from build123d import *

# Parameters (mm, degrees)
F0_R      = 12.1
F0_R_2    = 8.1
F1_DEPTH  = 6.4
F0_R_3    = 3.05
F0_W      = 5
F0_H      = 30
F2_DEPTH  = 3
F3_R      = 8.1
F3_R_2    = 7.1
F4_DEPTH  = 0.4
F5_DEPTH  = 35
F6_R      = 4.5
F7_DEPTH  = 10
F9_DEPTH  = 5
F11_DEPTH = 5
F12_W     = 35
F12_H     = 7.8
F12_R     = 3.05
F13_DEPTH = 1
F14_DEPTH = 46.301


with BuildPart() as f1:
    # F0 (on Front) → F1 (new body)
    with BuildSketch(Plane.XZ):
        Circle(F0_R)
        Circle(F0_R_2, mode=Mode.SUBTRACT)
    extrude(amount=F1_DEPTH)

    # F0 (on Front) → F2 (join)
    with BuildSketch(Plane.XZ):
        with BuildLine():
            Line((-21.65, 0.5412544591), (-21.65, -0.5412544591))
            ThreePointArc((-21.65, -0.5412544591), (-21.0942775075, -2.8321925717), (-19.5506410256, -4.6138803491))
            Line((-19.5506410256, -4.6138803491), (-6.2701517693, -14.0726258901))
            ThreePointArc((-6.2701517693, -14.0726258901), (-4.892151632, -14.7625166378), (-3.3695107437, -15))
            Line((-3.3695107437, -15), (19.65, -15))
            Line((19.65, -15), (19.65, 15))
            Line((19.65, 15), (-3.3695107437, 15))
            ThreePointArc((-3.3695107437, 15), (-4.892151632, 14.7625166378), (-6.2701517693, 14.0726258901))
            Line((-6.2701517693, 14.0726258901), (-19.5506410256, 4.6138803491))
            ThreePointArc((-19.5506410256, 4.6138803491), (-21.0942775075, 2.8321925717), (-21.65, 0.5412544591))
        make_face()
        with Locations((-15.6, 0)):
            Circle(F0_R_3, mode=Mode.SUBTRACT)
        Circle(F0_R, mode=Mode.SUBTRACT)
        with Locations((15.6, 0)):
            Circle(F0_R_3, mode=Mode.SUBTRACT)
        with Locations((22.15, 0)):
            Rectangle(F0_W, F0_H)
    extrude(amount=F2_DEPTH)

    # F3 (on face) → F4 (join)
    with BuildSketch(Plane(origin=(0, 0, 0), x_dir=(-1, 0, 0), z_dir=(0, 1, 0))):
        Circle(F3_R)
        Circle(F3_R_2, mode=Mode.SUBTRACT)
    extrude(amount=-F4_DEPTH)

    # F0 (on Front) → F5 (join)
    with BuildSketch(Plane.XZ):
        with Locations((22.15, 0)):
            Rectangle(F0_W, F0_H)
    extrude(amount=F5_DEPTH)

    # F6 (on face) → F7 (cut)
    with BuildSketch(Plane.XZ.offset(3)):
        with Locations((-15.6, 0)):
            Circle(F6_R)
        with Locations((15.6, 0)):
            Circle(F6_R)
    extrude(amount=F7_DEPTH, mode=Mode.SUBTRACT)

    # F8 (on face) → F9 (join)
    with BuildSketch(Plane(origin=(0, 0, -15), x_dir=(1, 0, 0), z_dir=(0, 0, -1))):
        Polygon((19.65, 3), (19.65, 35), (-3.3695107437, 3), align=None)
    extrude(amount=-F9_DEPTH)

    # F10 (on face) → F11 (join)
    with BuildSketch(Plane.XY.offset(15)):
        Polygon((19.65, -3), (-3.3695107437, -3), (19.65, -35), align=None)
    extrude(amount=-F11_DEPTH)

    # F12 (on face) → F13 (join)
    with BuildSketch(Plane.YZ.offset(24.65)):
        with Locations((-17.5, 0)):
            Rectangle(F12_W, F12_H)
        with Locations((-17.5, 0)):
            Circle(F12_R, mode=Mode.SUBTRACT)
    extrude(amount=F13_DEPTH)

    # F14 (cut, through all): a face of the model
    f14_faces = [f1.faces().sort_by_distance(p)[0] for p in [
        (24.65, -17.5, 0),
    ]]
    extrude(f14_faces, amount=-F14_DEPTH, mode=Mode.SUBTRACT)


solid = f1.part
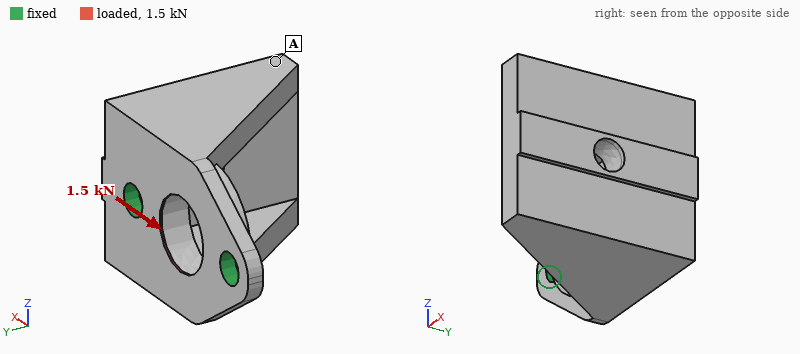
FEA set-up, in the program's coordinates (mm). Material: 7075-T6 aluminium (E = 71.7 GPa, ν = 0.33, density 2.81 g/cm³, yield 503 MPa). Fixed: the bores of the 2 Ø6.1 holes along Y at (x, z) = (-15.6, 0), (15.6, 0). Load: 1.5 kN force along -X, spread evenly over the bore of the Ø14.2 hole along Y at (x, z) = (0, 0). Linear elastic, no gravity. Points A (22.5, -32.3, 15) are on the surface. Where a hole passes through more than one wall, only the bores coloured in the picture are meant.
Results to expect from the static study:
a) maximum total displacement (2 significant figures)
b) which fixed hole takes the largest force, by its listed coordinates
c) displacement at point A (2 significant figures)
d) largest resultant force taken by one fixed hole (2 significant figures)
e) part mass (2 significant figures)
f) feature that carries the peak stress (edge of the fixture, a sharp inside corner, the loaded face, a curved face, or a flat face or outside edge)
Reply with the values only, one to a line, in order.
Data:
6.5 µm
(15.6, 0)
1.2 µm
810 N
34 g
the loaded face
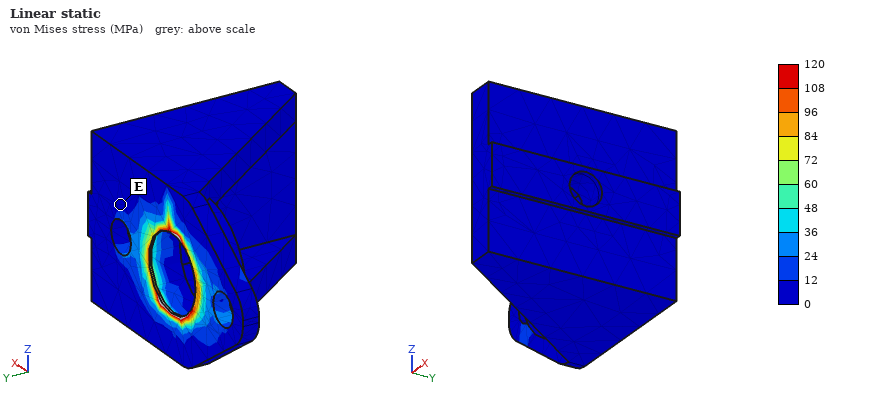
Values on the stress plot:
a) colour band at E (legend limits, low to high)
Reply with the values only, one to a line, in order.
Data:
0 to 12 MPa
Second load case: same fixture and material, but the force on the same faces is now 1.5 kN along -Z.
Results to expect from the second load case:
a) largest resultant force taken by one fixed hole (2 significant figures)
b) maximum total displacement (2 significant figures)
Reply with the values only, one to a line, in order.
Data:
760 N
14 µm
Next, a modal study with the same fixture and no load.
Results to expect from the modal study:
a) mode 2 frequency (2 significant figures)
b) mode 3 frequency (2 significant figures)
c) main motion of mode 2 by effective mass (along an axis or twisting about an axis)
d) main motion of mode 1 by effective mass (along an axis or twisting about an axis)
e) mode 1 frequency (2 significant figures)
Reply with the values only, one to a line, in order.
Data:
5500 Hz
10 kHz
along X
along Z
3000 Hz
